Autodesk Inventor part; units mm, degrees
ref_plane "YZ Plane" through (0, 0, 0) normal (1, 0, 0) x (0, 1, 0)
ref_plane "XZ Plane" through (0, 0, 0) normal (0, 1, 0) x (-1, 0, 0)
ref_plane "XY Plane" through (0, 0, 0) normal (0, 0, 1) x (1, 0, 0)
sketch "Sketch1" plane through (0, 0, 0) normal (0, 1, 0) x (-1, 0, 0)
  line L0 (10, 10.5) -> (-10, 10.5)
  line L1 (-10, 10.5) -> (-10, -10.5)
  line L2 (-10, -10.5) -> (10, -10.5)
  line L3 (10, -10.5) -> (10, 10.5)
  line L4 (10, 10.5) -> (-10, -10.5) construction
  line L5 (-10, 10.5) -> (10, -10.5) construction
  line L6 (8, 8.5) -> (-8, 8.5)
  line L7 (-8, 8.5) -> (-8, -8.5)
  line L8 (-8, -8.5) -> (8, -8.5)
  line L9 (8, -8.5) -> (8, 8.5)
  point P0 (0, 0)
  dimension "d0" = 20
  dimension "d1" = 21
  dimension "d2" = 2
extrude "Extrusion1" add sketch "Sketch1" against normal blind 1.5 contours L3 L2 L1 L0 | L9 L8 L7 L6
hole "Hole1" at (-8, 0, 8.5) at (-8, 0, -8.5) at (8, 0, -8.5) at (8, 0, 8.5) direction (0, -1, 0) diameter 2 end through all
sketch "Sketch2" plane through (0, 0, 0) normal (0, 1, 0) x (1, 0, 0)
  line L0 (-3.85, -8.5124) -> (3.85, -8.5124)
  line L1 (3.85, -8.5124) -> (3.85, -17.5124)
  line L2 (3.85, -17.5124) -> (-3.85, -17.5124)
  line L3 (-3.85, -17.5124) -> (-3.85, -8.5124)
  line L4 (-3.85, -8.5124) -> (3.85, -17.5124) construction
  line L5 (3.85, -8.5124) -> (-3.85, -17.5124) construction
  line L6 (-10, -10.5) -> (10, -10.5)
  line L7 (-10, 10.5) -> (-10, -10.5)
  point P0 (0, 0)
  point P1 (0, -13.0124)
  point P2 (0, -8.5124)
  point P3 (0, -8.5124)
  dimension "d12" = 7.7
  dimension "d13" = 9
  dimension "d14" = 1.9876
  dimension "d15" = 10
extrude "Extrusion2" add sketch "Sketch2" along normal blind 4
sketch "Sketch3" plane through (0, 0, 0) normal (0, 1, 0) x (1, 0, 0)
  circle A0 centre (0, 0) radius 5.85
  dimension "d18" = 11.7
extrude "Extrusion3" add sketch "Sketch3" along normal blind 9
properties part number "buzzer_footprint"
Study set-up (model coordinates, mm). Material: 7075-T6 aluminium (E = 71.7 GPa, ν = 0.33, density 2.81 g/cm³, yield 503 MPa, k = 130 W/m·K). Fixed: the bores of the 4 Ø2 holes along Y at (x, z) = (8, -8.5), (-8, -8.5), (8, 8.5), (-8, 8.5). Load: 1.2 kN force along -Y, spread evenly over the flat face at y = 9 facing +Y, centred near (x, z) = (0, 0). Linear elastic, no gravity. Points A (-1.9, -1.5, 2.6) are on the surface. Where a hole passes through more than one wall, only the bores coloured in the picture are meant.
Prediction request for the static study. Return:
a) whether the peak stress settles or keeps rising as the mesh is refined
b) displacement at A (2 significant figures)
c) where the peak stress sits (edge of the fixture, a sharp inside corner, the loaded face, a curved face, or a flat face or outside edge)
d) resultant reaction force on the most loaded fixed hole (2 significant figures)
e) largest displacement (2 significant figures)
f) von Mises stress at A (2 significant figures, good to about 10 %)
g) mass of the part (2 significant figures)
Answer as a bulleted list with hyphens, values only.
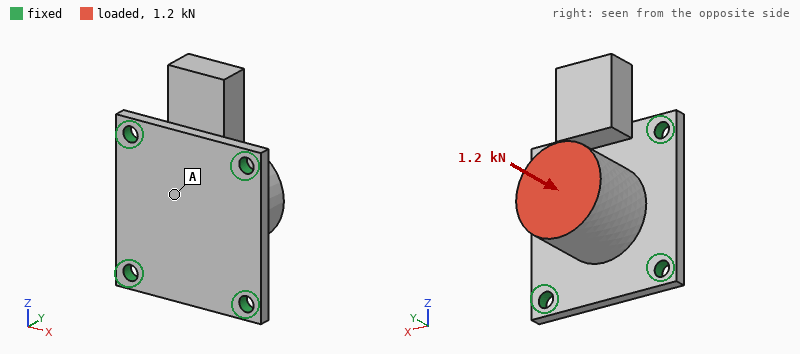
- keeps rising
- 43 µm
- edge of the fixture
- 320 N
- 51 µm
- 42 MPa
- 5.2 g
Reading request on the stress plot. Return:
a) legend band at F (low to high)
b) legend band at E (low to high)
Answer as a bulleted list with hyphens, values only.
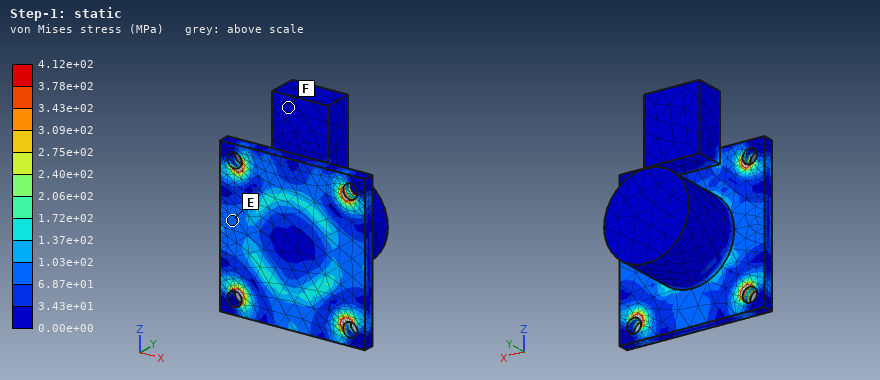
- 0.00e+00 to 3.43e+01 MPa
- 6.87e+01 to 1.03e+02 MPa
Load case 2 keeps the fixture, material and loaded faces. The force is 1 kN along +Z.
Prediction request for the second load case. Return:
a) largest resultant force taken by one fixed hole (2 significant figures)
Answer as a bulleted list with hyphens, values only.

- 460 N
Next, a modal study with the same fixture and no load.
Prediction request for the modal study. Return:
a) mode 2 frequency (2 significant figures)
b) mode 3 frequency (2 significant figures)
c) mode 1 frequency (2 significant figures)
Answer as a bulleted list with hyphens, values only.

- 14 kHz
- 14 kHz
- 8000 Hz
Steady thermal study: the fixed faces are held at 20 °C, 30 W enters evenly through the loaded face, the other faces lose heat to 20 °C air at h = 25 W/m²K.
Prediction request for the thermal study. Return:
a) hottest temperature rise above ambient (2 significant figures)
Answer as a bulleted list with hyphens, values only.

- 51 K
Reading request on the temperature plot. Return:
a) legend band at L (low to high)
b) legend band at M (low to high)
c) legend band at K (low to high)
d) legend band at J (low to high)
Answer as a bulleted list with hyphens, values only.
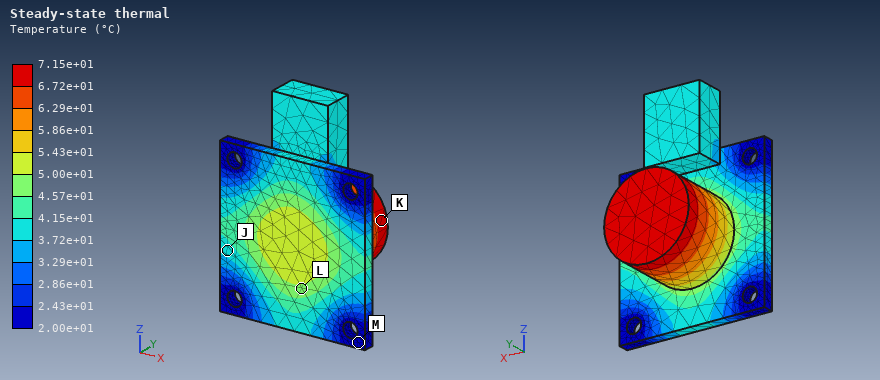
- 4.57e+01 to 5.00e+01 °C
- 2.00e+01 to 2.43e+01 °C
- 6.72e+01 to 7.15e+01 °C
- 3.72e+01 to 4.15e+01 °C
